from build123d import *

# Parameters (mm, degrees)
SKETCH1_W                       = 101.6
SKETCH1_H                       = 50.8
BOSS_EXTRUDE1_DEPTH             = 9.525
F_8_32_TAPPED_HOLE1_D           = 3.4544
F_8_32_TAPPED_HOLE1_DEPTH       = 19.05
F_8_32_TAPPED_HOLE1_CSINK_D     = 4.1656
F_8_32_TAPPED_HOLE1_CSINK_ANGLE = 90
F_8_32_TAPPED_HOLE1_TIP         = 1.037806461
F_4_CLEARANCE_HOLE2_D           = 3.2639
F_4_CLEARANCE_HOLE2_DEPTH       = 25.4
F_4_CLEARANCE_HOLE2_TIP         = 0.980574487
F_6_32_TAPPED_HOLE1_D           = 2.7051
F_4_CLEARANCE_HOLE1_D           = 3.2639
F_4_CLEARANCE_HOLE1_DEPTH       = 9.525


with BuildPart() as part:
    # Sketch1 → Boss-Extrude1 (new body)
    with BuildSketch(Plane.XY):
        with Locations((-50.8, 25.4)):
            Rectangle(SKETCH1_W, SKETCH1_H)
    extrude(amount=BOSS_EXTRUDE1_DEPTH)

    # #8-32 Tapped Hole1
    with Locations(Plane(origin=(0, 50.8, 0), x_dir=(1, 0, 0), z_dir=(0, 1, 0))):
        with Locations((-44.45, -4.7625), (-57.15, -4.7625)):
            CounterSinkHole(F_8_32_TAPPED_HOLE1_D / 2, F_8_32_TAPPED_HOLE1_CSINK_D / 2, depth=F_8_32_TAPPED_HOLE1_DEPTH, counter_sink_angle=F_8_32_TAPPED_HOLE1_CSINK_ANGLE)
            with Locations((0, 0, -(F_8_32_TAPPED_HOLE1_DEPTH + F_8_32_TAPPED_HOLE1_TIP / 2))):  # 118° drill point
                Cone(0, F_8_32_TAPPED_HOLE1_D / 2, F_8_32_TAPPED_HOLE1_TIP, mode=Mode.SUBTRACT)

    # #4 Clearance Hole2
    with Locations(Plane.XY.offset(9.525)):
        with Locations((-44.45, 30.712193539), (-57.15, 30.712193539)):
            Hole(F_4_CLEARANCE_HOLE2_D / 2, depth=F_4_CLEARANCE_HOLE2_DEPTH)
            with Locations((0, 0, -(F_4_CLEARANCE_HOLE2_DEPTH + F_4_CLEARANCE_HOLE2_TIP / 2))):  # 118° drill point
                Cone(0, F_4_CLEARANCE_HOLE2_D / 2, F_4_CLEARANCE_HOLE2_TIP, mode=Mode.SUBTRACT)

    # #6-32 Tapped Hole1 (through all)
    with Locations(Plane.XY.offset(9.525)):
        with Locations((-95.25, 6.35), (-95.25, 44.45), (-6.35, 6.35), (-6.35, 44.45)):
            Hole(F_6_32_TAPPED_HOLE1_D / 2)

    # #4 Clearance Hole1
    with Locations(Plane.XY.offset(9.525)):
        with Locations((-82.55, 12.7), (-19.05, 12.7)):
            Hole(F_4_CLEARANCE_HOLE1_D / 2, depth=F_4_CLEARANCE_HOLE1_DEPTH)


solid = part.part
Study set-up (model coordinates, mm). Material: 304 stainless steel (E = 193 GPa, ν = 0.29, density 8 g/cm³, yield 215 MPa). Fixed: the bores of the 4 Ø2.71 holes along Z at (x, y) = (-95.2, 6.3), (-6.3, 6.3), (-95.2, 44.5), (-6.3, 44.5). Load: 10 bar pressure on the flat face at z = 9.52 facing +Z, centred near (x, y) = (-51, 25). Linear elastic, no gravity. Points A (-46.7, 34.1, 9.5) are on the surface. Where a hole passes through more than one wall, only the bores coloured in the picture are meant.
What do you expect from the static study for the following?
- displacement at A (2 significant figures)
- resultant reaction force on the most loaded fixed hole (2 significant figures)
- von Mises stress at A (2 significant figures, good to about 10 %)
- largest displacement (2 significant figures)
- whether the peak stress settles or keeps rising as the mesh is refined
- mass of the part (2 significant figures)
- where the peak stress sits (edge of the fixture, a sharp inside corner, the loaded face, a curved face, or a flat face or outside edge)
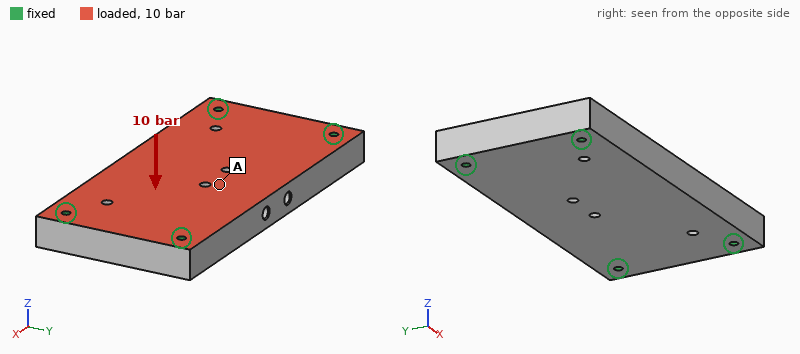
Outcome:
19 µm
1.3 kN
28 MPa
20 µm
keeps rising
390 g
edge of the fixture
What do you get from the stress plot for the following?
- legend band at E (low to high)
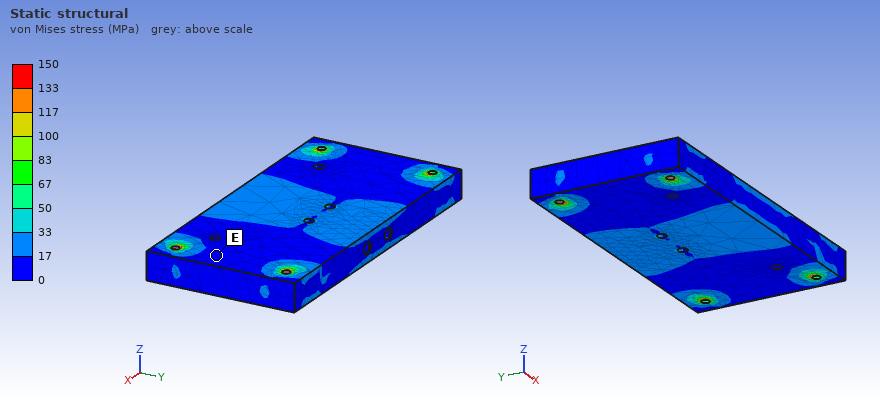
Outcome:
0 to 17 MPa
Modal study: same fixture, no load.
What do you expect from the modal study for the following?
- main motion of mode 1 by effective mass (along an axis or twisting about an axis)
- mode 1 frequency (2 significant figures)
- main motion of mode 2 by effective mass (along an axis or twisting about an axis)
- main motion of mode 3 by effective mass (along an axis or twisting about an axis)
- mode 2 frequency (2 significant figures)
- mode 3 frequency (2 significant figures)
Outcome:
along Z
4700 Hz
twisting about X
twisting about Y
7900 Hz
12 kHz
